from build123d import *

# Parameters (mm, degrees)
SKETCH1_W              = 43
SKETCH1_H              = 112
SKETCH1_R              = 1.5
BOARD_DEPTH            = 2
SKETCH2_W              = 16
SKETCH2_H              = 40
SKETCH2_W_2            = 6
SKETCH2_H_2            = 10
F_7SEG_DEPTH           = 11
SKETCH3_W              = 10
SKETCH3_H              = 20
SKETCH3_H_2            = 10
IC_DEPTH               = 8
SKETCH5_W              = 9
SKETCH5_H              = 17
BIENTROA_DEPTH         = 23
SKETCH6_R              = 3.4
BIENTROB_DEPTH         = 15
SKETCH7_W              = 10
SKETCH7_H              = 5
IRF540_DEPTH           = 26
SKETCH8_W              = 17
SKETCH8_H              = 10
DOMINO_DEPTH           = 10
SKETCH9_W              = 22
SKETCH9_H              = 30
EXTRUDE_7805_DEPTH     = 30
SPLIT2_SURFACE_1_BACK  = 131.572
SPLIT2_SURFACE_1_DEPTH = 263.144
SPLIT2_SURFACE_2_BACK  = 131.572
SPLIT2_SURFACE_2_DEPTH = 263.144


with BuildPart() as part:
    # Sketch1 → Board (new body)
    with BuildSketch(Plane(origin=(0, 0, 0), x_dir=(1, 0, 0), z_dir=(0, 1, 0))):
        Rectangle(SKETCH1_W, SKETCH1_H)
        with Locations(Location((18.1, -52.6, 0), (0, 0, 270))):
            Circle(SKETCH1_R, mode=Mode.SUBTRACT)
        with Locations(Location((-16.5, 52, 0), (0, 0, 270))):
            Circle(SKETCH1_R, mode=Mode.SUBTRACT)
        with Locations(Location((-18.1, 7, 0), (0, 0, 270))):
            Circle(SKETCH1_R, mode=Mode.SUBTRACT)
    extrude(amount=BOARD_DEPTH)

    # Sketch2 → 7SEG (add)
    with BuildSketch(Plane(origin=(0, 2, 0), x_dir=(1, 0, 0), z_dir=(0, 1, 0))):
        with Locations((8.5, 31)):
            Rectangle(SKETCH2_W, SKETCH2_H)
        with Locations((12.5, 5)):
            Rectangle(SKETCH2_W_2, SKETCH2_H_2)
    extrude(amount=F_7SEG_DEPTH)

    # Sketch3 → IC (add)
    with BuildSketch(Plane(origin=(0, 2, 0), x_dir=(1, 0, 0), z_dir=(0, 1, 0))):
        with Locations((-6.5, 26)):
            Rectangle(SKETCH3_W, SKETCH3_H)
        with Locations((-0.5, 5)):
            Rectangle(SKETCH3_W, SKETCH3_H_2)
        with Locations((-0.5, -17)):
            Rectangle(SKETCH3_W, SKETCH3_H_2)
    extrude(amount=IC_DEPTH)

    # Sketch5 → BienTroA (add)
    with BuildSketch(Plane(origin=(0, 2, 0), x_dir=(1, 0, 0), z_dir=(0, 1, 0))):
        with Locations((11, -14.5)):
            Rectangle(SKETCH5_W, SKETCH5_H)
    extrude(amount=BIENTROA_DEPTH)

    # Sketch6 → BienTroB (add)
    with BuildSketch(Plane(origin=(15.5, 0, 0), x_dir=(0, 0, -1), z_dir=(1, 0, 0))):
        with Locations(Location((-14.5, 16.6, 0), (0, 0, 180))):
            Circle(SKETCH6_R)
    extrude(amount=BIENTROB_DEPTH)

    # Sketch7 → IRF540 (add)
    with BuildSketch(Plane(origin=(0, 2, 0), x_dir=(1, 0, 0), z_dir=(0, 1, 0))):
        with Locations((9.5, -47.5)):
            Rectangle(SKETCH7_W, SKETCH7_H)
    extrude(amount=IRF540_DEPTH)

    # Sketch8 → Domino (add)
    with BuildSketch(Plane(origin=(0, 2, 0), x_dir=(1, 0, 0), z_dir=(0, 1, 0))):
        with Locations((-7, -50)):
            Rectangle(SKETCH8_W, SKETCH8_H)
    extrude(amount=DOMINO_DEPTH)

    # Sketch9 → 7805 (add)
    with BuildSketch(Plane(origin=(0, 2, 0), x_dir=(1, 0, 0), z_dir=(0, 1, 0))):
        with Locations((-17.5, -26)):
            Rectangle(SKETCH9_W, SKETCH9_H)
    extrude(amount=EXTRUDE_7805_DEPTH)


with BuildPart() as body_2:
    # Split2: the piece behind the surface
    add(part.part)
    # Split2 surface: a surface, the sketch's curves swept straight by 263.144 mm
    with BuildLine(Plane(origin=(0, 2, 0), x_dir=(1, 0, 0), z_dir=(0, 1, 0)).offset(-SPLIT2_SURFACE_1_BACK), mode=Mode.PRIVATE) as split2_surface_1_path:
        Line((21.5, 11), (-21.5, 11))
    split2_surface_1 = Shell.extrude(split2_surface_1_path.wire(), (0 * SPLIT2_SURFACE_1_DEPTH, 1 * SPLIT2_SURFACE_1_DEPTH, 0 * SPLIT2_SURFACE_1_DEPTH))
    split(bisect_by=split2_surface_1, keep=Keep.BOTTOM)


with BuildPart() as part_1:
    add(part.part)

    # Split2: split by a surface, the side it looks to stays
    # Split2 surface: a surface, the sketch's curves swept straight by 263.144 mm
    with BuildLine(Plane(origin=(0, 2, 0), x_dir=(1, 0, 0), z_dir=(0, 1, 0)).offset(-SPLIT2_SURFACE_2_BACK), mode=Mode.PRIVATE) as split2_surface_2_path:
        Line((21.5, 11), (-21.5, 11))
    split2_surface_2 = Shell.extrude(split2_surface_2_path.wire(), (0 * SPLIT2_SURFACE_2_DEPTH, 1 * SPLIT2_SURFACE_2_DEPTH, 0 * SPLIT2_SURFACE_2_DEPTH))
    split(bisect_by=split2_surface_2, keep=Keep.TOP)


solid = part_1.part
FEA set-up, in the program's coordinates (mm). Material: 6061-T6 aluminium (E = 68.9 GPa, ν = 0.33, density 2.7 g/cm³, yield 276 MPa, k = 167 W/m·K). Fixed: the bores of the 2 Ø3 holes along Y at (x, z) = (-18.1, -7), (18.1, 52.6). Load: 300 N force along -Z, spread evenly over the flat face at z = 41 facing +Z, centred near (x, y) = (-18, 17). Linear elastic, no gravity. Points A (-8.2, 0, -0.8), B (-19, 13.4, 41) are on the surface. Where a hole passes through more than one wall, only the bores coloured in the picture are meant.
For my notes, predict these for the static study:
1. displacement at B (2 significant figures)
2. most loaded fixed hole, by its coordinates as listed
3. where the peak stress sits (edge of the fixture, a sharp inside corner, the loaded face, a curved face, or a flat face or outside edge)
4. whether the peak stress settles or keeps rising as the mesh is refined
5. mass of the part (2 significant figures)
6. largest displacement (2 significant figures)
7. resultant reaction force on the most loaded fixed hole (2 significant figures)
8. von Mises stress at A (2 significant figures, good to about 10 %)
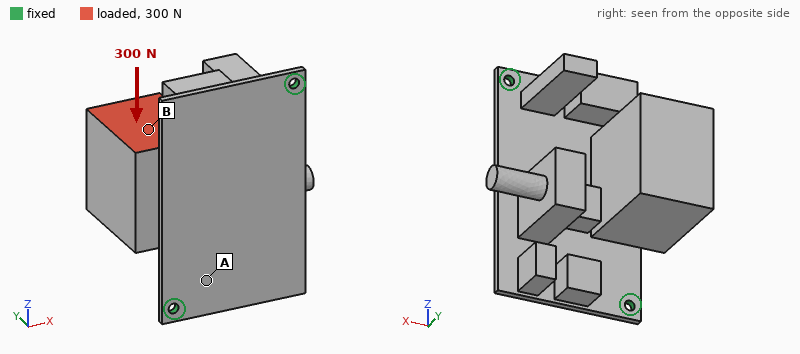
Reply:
0.37 mm
(-18.1, -7)
edge of the fixture
keeps rising
94 g
0.59 mm
210 N
22 MPa
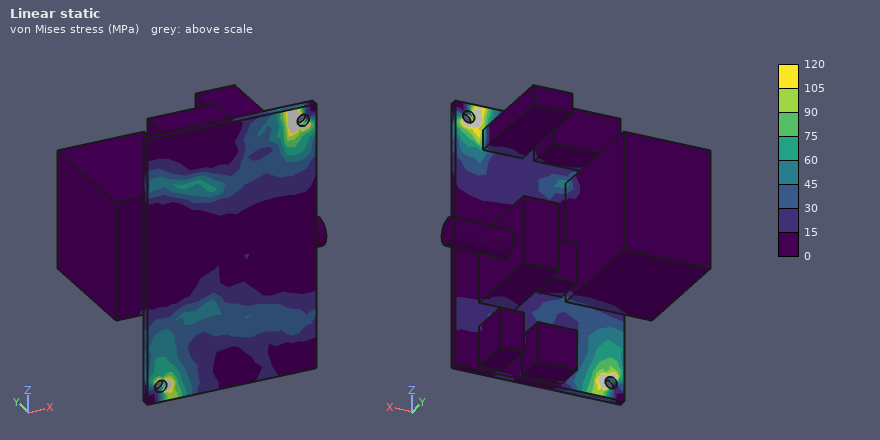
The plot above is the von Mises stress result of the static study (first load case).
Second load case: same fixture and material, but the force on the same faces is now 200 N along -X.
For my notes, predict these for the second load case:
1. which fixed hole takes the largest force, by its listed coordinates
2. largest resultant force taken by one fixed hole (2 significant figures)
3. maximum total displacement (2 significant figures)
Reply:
(18.1, 52.6)
160 N
0.71 mm
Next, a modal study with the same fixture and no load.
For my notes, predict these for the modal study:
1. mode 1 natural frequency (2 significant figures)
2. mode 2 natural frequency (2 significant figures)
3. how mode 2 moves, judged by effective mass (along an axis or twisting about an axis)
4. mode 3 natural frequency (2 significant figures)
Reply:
320 Hz
850 Hz
along Y
1200 Hz
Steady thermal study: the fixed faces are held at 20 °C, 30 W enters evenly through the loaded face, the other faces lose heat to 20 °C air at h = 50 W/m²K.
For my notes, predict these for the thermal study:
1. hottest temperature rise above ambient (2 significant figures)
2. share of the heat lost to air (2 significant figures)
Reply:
38 K
49 %
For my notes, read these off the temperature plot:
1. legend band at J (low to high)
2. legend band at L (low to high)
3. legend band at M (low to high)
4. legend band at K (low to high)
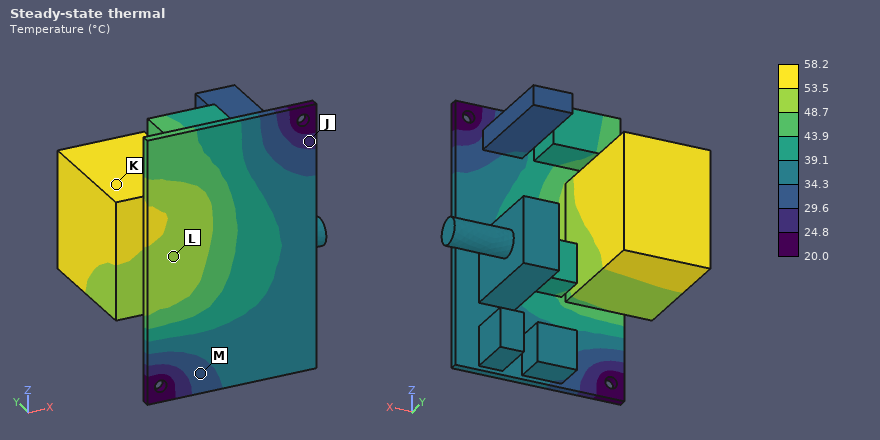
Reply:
24.8 to 29.6 °C
48.7 to 53.5 °C
29.6 to 34.3 °C
53.5 to 58.2 °C
